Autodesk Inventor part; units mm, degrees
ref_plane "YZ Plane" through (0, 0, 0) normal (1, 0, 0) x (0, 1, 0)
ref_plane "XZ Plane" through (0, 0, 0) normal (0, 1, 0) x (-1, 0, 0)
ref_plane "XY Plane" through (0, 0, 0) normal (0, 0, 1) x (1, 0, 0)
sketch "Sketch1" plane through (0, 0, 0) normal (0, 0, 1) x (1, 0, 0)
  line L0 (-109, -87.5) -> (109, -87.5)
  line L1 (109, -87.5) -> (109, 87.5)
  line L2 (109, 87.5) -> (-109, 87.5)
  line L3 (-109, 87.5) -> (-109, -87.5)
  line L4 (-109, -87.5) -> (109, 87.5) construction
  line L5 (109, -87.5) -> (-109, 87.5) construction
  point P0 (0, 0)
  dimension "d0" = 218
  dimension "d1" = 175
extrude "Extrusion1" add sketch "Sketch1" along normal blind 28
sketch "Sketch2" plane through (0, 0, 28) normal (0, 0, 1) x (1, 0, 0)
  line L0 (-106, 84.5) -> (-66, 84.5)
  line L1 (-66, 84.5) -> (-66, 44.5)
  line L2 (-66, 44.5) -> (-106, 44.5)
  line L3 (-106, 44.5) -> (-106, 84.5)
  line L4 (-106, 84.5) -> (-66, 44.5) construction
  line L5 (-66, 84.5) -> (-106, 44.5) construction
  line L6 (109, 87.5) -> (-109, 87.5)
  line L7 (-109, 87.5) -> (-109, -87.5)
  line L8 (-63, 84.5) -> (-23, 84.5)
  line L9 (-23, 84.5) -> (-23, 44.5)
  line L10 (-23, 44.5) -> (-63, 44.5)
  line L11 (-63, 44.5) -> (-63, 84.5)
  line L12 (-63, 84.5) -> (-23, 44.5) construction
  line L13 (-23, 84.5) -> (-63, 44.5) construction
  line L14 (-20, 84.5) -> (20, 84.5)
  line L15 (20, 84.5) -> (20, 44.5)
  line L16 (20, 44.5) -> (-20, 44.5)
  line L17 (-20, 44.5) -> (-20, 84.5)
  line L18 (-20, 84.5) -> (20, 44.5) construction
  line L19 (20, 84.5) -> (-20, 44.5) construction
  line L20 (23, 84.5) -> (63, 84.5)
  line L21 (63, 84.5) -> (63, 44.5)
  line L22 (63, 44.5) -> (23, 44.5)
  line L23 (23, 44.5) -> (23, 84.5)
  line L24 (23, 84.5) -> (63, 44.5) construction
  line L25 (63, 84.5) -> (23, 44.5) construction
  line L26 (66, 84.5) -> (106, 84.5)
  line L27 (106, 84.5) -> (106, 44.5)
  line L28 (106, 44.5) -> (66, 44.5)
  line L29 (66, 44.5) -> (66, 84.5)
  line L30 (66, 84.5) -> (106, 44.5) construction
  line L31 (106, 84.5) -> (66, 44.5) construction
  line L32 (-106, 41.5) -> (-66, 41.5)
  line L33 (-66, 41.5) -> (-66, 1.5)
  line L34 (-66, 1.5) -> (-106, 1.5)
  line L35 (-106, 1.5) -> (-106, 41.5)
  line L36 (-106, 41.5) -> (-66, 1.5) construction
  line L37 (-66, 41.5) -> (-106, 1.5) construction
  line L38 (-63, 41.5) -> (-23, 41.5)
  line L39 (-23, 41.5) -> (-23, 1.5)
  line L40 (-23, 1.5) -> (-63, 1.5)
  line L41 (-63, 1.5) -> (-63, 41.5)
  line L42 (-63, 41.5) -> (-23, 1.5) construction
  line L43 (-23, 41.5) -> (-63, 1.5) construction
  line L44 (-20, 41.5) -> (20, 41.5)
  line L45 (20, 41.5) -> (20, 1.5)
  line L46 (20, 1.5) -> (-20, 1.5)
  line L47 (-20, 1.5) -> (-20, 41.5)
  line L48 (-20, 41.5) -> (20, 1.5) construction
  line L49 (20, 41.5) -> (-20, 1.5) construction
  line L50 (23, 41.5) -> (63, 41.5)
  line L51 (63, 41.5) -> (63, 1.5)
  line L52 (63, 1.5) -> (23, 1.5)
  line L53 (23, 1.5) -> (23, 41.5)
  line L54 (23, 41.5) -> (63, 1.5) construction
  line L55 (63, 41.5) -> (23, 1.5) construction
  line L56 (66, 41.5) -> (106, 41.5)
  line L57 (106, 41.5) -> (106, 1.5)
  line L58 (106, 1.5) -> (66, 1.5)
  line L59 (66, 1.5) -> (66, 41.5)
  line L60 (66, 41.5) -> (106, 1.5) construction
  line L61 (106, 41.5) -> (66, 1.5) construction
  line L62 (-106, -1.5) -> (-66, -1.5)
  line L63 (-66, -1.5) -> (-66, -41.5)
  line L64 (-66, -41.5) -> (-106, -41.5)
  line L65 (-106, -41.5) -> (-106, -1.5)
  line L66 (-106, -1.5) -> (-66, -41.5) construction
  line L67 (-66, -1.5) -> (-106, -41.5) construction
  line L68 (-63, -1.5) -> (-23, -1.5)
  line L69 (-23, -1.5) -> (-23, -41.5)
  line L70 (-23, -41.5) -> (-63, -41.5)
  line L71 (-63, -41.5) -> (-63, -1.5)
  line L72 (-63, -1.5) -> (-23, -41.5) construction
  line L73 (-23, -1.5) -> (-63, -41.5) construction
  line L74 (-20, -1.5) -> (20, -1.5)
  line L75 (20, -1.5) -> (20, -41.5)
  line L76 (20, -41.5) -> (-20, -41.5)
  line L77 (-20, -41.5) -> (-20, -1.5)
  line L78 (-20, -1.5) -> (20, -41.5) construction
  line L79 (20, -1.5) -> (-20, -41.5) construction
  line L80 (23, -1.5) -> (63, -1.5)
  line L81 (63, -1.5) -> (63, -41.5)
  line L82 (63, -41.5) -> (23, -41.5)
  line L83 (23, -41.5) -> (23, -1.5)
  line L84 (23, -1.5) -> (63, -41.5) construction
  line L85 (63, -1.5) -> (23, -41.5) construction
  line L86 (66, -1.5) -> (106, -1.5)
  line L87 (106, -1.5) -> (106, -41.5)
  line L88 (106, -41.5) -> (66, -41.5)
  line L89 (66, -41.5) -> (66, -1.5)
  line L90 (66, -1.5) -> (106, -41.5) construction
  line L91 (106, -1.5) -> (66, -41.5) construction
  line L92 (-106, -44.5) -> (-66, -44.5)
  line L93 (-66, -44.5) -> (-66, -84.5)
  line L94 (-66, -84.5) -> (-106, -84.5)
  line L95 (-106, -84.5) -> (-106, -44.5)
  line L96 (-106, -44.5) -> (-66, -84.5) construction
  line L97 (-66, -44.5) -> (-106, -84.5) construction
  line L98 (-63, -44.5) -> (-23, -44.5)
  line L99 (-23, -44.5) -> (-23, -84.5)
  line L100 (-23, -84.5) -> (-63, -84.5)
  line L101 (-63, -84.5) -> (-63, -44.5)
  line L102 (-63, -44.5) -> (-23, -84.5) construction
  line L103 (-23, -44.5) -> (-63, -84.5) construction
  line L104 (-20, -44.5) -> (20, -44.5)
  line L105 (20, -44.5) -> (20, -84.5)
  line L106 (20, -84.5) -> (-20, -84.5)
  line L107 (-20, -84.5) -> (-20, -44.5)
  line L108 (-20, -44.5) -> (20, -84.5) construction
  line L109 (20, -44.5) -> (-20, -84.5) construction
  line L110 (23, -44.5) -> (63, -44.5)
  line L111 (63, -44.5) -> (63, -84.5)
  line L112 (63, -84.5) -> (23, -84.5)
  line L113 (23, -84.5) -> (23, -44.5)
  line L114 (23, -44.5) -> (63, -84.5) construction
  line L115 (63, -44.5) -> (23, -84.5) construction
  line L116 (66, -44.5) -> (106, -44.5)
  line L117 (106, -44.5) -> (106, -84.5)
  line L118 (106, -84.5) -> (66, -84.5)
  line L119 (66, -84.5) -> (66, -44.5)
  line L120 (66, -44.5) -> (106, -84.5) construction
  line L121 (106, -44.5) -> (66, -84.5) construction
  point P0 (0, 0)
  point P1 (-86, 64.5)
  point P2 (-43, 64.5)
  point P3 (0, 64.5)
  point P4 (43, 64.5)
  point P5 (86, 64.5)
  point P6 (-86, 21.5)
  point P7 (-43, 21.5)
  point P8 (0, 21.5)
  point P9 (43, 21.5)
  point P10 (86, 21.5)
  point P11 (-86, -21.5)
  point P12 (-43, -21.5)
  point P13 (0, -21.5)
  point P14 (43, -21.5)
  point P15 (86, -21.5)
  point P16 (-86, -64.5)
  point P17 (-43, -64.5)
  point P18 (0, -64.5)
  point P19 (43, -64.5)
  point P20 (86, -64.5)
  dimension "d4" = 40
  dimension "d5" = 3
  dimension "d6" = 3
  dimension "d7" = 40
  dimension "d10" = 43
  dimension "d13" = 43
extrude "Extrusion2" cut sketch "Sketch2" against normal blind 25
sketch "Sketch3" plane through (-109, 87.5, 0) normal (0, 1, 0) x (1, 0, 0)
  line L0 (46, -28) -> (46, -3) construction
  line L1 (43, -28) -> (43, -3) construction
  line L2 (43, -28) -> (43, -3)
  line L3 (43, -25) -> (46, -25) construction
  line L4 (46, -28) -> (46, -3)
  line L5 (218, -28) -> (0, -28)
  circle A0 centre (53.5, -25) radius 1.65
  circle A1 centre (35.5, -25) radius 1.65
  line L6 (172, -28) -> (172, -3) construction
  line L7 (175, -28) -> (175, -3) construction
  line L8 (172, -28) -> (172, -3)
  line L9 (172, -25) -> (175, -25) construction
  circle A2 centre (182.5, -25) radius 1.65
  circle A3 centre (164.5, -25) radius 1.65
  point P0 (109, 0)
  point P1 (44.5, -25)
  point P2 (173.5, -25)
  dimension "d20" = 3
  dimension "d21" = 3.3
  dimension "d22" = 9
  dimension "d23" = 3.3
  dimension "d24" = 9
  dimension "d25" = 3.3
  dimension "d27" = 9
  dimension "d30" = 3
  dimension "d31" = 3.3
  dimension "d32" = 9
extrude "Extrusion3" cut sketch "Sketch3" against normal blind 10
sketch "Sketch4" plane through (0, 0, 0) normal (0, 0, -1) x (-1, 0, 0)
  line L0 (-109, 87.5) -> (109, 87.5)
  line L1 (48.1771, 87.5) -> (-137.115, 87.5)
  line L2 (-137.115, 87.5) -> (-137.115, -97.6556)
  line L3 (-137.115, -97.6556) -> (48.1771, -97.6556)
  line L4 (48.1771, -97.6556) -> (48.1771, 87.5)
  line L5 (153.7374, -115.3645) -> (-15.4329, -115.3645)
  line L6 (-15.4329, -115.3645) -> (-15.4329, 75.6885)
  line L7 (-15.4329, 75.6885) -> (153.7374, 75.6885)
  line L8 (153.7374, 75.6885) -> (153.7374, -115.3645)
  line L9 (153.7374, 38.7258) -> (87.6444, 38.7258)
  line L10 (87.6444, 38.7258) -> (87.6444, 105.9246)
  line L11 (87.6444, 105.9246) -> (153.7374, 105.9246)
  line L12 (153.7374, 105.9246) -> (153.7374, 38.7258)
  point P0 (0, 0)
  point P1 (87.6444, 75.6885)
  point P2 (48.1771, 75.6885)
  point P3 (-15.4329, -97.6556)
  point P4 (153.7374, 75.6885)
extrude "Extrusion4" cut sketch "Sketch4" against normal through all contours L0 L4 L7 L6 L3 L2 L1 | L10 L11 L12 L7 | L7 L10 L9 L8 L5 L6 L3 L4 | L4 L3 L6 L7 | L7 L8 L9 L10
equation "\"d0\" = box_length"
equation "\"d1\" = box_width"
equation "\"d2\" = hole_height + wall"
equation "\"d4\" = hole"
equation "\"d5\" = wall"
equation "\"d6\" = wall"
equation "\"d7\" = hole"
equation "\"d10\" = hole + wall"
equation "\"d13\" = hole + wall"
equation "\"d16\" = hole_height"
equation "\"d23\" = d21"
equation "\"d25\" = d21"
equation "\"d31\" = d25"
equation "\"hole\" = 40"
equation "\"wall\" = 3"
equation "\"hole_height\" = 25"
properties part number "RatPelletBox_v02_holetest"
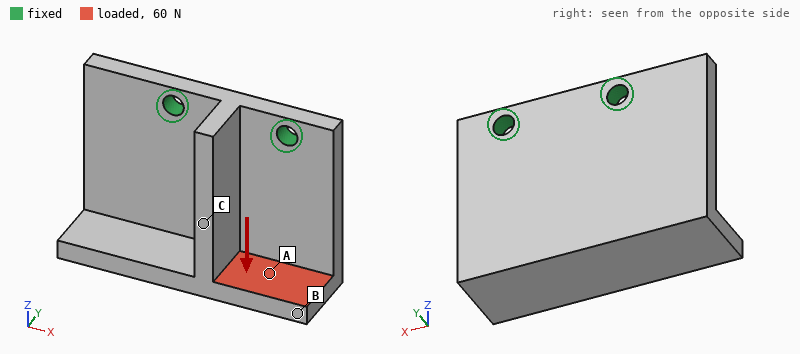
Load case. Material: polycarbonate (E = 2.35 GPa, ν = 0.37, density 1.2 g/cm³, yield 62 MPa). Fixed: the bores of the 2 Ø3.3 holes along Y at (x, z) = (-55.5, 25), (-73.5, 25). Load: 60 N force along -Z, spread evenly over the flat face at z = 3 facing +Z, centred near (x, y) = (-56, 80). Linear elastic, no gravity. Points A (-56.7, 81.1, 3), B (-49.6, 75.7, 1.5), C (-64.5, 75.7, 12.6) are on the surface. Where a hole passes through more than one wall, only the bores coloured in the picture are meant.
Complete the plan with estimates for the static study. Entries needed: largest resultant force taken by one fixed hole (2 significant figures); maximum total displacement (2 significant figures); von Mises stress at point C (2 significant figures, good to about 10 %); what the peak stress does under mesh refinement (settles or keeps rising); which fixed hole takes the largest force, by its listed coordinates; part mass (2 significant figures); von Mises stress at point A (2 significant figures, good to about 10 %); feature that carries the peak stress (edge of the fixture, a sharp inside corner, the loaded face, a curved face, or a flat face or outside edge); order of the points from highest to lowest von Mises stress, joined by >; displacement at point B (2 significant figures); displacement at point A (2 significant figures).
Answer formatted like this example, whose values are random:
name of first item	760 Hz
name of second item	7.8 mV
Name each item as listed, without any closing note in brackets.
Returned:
largest resultant force taken by one fixed hole	57 N
maximum total displacement	0.48 mm
von Mises stress at point C	3.2 MPa
what the peak stress does under mesh refinement	keeps rising
which fixed hole takes the largest force, by its listed coordinates	(-55.5, 25)
part mass	6.0 g
von Mises stress at point A	5.3 MPa
feature that carries the peak stress	edge of the fixture
order of the points from highest to lowest von Mises stress, joined by >	A > C > B
displacement at point B	0.43 mm
displacement at point A	0.27 mm
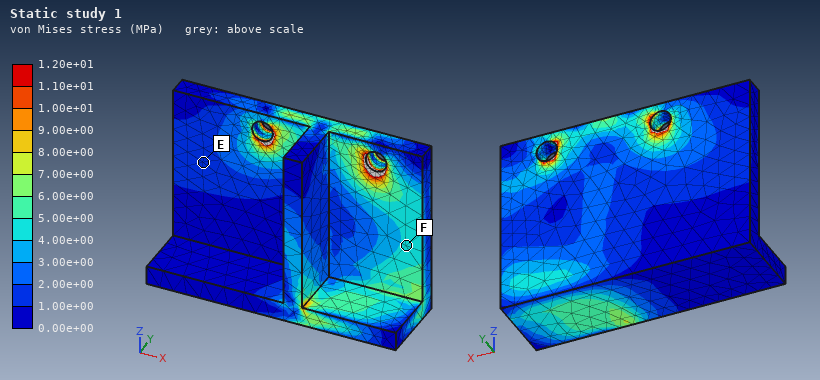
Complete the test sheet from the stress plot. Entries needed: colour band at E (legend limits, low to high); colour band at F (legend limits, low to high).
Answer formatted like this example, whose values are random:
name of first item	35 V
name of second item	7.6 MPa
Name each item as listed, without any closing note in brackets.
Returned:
colour band at E	1.00e+00 to 2.00e+00 MPa
colour band at F	4.00e+00 to 5.00e+00 MPa
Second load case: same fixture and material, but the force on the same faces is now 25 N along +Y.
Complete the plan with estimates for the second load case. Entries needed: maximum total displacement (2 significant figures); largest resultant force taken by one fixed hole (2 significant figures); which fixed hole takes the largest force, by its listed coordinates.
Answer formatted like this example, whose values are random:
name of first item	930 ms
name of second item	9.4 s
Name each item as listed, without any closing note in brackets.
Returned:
maximum total displacement	0.56 mm
largest resultant force taken by one fixed hole	24 N
which fixed hole takes the largest force, by its listed coordinates	(-55.5, 25)
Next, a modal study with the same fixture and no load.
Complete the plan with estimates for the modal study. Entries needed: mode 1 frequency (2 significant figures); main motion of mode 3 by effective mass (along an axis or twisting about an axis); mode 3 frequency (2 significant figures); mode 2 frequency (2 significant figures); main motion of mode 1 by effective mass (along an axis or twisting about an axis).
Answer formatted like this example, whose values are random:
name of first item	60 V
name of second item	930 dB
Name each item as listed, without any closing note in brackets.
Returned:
mode 1 frequency	780 Hz
main motion of mode 3 by effective mass	along X
mode 3 frequency	3200 Hz
mode 2 frequency	1300 Hz
main motion of mode 1 by effective mass	along Y
